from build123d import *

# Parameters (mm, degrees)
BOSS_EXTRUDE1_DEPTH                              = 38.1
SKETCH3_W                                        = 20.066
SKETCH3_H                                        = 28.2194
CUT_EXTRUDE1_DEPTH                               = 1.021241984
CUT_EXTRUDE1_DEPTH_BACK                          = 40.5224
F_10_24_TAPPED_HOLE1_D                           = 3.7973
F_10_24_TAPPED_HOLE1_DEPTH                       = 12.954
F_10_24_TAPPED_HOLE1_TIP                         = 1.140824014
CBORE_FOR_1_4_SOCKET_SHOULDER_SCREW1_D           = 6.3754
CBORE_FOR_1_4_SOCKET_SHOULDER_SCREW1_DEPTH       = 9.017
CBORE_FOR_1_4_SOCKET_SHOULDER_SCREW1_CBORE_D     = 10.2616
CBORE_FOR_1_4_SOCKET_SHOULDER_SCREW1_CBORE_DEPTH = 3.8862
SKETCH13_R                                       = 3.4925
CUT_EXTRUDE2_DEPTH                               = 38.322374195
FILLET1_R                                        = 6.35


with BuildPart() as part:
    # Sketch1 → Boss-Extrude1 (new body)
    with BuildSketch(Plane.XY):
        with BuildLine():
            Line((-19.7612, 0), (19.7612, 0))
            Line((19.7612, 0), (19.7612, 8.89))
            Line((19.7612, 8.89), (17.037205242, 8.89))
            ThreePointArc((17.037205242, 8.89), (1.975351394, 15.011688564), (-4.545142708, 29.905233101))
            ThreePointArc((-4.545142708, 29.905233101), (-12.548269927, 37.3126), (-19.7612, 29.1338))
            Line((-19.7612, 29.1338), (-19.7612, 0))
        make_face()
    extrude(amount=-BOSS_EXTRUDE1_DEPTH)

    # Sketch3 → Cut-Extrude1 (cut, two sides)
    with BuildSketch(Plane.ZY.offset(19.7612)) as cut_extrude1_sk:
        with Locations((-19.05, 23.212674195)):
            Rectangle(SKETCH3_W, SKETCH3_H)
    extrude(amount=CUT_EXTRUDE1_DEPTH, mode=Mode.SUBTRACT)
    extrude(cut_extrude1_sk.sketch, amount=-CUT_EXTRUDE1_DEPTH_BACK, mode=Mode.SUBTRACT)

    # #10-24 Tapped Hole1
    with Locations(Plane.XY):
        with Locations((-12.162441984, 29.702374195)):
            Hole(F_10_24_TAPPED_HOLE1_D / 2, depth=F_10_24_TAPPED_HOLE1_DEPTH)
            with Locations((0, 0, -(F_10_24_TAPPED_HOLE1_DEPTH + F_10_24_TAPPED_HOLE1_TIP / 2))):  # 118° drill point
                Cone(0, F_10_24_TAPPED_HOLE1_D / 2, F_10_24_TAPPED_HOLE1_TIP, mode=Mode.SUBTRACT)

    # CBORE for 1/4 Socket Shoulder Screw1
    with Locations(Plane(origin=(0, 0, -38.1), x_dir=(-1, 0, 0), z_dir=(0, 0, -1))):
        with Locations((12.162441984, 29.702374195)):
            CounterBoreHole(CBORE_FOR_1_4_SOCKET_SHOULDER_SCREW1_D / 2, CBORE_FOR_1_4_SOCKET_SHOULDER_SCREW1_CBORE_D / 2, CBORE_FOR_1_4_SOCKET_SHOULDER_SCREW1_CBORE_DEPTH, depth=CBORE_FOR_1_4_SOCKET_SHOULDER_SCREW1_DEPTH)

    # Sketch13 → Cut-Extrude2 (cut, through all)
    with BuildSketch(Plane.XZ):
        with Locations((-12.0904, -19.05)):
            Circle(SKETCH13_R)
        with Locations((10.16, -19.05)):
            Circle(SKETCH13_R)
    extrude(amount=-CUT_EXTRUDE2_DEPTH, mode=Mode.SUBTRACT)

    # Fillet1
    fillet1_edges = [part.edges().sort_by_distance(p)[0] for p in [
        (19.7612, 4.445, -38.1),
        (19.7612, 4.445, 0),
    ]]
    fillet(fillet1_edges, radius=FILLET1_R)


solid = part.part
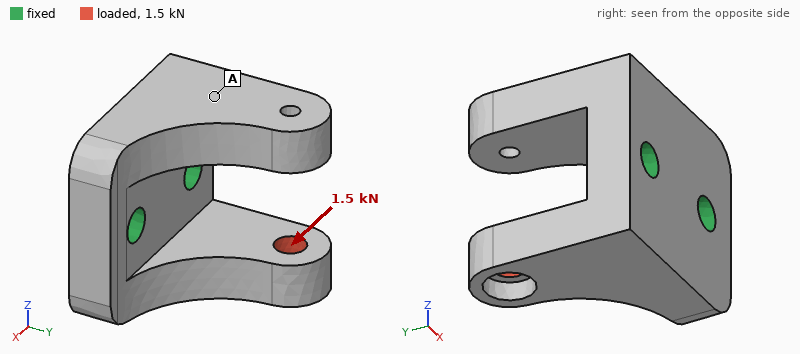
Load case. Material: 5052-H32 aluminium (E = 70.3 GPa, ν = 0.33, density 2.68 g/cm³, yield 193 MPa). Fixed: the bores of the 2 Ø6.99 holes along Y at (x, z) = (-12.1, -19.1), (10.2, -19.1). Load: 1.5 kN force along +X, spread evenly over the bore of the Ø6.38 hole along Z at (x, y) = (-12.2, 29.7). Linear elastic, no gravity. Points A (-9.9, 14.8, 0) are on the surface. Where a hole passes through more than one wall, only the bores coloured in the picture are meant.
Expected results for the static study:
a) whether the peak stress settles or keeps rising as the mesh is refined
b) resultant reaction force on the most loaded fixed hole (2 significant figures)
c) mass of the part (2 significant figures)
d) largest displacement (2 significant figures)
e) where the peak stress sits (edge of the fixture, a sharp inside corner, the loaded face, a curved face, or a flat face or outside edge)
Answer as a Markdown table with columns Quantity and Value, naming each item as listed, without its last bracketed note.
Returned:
| Quantity | Value |
|---|---|
| whether the peak stress settles or keeps rising as the mesh is refined | keeps rising |
| resultant reaction force on the most loaded fixed hole | 1.7 kN |
| mass of the part | 57 g |
| largest displacement | 75 µm |
| where the peak stress sits | edge of the fixture |
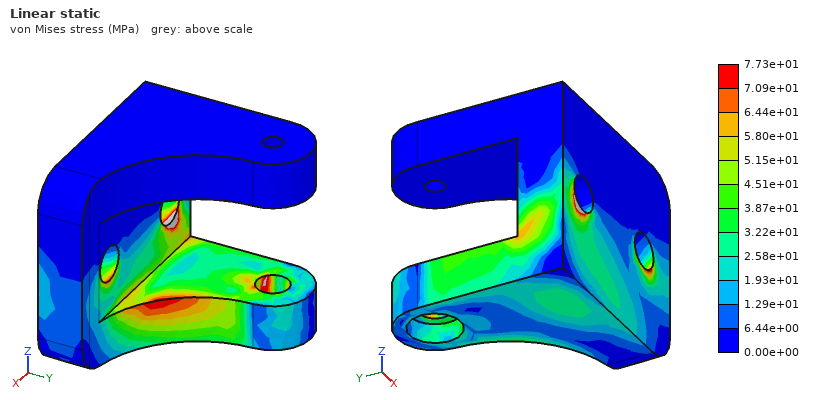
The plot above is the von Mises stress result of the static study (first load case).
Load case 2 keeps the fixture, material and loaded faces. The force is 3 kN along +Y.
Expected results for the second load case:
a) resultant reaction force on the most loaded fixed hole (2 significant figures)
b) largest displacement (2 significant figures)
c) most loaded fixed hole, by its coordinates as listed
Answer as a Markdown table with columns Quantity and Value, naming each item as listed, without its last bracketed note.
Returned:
| Quantity | Value |
|---|---|
| resultant reaction force on the most loaded fixed hole | 2.7 kN |
| largest displacement | 51 µm |
| most loaded fixed hole, by its coordinates as listed | (-12.1, -19.1) |
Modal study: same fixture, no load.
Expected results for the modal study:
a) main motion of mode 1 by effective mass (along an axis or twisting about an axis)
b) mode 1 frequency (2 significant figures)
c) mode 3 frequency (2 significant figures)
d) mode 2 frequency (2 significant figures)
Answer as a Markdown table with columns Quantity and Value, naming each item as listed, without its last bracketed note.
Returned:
| Quantity | Value |
|---|---|
| main motion of mode 1 by effective mass | along Z |
| mode 1 frequency | 6300 Hz |
| mode 3 frequency | 11 kHz |
| mode 2 frequency | 6900 Hz |
